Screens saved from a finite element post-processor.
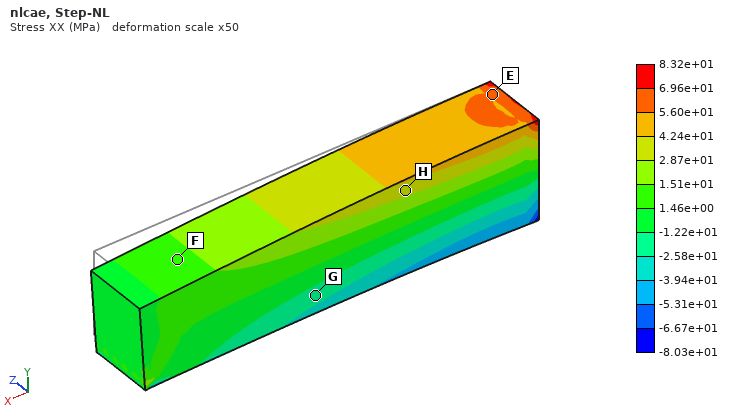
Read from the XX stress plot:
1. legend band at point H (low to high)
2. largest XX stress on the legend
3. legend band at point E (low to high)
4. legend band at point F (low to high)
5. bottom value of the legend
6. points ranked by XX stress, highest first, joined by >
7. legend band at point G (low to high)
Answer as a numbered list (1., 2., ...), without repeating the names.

1. 2.87e+01 to 4.24e+01 MPa
2. 8.32e+01 MPa
3. 5.60e+01 to 6.96e+01 MPa
4. 1.46e+00 to 1.51e+01 MPa
5. -8.03e+01 MPa
6. E > H > F > G
7. -2.58e+01 to -1.22e+01 MPa
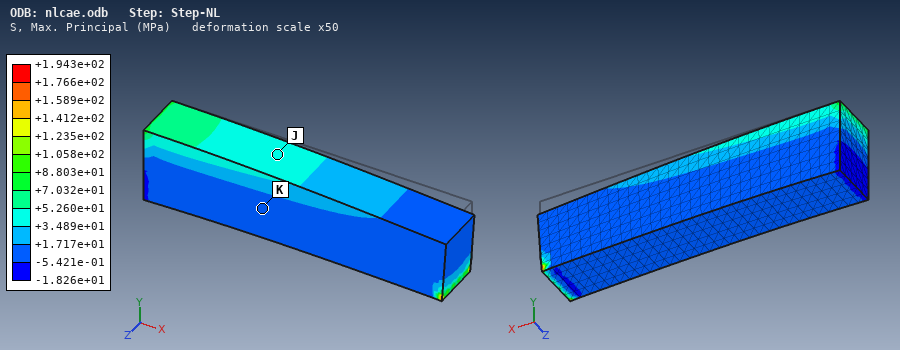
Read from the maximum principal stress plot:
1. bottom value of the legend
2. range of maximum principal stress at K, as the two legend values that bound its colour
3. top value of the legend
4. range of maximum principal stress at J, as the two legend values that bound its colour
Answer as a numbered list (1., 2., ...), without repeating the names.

1. -1.826e+01 MPa
2. -5.421e-01 to +1.717e+01 MPa
3. +1.943e+02 MPa
4. +3.489e+01 to +5.260e+01 MPa
